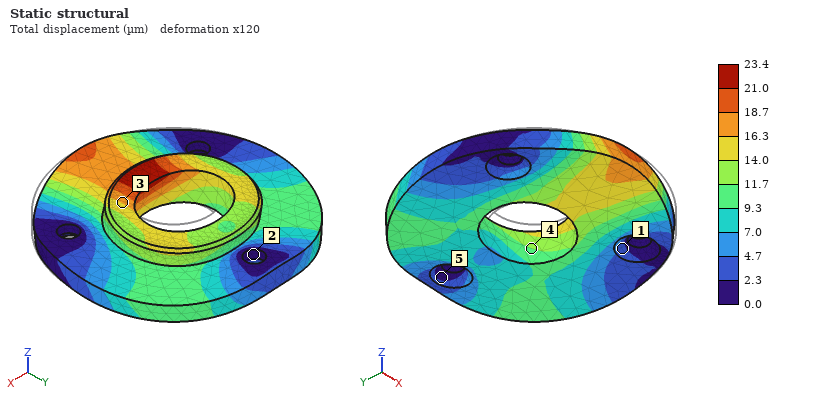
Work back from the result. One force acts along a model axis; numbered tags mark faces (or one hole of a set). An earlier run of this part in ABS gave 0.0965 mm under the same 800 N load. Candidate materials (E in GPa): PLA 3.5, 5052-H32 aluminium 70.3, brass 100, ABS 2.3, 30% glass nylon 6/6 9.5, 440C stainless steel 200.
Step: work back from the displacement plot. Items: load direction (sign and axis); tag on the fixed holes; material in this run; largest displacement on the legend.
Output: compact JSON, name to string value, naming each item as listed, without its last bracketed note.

{"load direction": "+Y", "tag on the fixed holes": "2", "material in this run": "30% glass nylon 6/6", "largest displacement on the legend": "23.4 µm"}
